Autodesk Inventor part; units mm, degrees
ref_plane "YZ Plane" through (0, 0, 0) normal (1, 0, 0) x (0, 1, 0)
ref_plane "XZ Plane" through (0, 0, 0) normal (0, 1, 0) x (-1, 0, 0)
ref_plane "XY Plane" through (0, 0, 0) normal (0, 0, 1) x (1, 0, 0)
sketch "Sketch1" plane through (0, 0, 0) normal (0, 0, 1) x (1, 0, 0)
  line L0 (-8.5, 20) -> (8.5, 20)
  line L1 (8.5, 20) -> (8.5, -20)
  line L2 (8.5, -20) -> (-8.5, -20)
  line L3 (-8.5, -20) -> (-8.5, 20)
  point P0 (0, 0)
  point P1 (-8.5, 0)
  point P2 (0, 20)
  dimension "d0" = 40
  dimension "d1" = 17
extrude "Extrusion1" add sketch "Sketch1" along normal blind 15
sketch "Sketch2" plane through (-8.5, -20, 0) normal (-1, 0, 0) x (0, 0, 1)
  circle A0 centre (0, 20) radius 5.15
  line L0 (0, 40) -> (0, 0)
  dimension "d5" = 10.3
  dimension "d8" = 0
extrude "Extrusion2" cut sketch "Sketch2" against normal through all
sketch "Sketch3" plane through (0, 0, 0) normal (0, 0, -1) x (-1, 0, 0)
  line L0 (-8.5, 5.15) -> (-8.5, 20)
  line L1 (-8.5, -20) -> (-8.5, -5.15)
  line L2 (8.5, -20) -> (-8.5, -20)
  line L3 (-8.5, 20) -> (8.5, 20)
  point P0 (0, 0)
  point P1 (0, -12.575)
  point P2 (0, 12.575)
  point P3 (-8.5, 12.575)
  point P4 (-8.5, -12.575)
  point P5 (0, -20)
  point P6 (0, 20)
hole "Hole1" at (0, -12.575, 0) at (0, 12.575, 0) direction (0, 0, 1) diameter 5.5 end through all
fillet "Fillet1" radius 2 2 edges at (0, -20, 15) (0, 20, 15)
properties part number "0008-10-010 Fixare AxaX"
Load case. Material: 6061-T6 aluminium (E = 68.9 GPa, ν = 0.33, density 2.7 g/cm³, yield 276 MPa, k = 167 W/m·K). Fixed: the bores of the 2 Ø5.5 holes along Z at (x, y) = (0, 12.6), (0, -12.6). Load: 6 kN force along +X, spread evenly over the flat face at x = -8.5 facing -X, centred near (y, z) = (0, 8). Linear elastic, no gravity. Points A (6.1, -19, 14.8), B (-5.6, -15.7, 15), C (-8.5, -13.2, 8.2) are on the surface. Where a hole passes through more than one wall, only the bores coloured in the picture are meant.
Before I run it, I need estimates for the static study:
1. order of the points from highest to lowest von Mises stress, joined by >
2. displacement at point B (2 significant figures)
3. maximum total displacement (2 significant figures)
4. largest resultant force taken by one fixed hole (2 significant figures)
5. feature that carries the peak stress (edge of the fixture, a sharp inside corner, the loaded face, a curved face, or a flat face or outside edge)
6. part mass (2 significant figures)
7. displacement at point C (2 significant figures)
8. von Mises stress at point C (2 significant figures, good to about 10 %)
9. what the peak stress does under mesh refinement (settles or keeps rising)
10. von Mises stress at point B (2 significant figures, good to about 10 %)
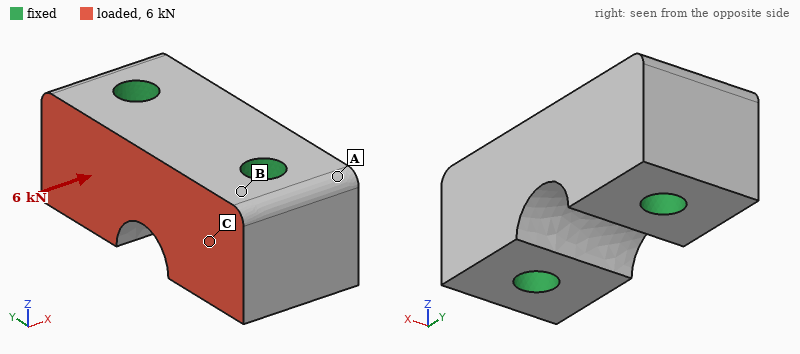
C > B > A
0.96 µm
3.4 µm
3.0 kN
edge of the fixture
24 g
1.1 µm
17 MPa
keeps rising
11 MPa
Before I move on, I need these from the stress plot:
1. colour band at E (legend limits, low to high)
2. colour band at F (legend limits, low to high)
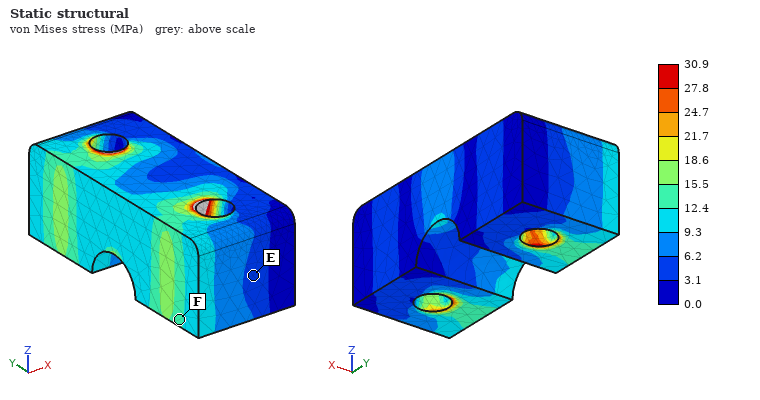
3.1 to 6.2 MPa
12.4 to 15.5 MPa
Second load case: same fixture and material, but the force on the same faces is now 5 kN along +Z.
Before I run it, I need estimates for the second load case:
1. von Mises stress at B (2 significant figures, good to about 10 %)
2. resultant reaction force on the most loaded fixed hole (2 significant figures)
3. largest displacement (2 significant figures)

15 MPa
2.5 kN
8.7 µm
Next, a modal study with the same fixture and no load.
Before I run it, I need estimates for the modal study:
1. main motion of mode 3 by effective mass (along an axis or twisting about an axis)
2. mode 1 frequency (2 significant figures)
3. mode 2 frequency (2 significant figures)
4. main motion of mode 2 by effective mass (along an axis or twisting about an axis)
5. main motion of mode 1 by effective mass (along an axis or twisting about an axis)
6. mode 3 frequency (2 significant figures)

twisting about Y
52 kHz
57 kHz
along Z
along X
65 kHz
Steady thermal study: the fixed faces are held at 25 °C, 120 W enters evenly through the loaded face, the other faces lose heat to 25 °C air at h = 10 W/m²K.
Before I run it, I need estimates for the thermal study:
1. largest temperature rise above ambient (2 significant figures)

13 K
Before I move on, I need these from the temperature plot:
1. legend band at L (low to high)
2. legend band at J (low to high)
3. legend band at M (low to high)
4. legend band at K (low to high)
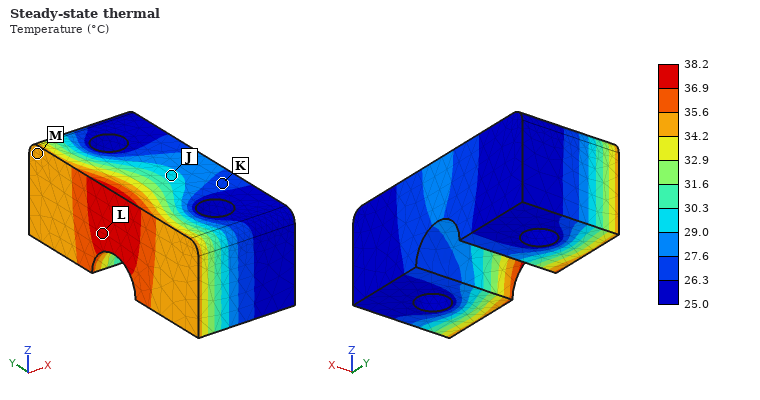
36.9 to 38.2 °C
29.0 to 30.3 °C
34.2 to 35.6 °C
26.3 to 27.6 °C
